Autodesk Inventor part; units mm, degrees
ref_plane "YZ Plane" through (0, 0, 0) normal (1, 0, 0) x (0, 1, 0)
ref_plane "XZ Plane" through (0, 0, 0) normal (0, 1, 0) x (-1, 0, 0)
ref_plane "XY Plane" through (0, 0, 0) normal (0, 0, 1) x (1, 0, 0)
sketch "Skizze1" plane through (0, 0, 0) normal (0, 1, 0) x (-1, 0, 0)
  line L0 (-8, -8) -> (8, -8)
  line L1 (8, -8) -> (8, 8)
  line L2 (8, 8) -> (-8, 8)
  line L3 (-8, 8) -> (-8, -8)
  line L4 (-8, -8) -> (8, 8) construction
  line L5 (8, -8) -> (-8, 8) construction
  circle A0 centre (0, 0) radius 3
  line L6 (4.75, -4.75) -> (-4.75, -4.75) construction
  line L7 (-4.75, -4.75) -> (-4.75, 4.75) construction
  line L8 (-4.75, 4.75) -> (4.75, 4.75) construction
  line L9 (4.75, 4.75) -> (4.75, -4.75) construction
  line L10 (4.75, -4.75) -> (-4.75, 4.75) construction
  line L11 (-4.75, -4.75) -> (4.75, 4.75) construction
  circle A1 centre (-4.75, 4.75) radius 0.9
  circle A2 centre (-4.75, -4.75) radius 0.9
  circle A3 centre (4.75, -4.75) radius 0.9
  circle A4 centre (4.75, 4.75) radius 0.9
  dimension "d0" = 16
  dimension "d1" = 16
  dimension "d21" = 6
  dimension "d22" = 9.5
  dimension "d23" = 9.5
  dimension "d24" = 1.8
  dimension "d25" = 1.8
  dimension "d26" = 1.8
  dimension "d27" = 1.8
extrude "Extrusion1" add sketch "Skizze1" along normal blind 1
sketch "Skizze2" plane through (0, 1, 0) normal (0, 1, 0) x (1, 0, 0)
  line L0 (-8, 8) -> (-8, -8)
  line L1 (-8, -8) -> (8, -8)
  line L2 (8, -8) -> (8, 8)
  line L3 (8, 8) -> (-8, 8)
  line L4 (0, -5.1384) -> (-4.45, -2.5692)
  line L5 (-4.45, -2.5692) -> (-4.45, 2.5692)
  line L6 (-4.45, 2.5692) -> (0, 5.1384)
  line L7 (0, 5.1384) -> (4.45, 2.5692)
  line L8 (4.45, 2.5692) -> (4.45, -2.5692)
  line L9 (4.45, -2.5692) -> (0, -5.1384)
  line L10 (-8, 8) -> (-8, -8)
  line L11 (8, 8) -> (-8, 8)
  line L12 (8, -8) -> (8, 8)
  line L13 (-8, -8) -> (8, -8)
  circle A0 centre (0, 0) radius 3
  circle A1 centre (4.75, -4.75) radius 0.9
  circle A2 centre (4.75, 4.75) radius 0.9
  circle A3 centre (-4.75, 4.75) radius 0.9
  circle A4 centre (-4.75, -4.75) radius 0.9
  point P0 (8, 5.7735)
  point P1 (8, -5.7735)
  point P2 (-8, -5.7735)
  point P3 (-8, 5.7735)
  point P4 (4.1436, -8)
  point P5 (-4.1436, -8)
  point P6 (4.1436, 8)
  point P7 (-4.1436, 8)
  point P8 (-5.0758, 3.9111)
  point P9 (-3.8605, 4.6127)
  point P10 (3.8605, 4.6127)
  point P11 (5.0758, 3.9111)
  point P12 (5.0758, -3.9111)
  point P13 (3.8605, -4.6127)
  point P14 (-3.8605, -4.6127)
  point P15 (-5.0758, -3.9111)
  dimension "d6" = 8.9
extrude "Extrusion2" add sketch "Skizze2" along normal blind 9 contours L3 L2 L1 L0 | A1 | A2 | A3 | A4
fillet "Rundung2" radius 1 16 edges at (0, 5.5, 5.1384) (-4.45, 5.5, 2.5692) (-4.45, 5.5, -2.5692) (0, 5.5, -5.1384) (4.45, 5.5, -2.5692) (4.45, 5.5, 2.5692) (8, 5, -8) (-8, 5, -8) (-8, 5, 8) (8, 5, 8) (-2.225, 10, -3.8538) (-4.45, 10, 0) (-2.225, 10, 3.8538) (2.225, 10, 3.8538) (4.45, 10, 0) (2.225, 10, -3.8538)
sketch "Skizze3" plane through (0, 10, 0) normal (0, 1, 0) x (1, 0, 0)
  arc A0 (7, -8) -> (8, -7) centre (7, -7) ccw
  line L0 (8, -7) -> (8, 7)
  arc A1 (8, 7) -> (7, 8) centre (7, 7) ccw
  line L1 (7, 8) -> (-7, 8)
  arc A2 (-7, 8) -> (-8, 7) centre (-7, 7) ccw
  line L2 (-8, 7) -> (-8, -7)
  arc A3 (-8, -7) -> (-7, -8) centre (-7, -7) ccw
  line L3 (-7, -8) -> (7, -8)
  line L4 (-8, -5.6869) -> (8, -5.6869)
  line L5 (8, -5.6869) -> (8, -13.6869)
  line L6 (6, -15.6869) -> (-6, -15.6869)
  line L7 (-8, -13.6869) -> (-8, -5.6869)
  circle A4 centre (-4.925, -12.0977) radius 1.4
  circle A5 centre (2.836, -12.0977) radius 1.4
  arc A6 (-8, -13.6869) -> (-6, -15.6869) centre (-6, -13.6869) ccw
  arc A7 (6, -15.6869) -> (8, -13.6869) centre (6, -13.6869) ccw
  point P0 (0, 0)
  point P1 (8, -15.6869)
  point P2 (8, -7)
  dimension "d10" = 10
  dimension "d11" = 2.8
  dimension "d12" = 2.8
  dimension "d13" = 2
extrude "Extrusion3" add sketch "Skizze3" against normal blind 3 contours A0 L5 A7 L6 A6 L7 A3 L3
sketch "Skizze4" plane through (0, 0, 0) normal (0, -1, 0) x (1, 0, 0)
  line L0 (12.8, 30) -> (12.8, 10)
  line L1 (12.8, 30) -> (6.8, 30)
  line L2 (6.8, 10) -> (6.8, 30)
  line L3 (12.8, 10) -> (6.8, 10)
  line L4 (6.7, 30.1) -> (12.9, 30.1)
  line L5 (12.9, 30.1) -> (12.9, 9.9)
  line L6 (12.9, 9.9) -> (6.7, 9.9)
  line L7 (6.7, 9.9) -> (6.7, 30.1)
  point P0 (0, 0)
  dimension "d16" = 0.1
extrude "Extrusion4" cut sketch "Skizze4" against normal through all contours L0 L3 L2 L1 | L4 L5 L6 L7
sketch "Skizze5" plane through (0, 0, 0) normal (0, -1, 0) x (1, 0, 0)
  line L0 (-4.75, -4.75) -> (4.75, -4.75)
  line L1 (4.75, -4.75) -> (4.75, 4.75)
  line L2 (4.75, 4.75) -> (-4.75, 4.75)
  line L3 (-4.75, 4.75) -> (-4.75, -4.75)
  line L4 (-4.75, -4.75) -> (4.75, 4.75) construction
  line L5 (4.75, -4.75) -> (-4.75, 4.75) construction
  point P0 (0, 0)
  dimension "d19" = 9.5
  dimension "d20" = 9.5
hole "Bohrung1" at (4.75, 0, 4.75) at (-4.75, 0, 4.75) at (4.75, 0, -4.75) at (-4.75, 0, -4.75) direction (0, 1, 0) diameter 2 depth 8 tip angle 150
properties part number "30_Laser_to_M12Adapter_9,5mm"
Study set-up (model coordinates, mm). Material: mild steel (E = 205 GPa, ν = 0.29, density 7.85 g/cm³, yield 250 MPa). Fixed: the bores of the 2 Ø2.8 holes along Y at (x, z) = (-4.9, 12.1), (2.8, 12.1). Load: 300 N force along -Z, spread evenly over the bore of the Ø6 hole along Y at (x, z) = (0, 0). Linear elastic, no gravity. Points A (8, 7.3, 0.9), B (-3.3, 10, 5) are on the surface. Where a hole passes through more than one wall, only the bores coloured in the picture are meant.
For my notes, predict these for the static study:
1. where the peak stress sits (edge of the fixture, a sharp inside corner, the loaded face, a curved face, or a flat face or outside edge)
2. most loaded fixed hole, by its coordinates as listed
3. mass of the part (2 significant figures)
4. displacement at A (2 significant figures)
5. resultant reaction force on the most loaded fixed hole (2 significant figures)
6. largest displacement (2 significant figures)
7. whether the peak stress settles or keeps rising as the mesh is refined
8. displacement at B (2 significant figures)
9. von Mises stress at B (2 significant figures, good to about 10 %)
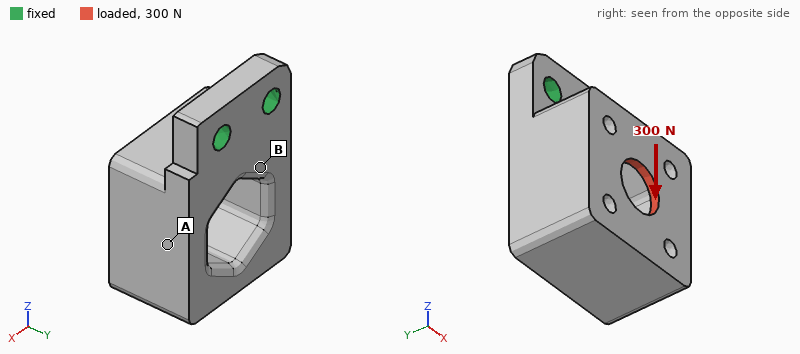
edge of the fixture
(2.8, 12.1)
17 g
14 µm
180 N
34 µm
keeps rising
6.9 µm
24 MPa
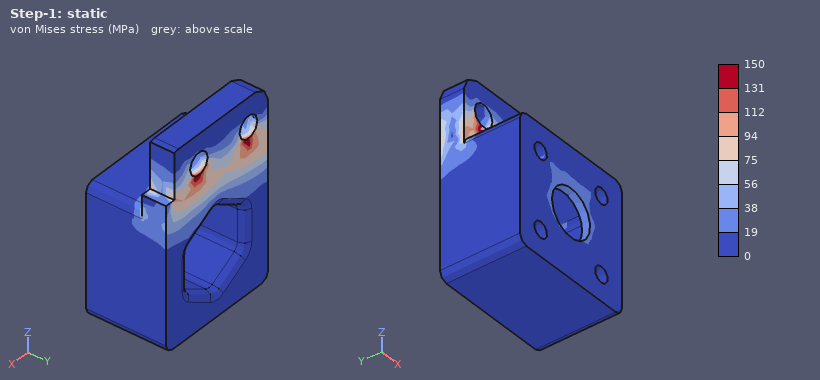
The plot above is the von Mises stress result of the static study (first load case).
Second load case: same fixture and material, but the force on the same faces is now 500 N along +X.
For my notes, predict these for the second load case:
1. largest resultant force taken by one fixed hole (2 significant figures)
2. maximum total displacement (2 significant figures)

750 N
12 µm
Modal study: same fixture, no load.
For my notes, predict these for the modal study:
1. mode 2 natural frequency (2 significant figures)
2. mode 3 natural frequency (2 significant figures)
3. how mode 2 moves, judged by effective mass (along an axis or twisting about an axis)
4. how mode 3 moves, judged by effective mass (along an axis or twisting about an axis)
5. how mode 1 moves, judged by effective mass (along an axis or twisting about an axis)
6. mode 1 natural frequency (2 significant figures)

12 kHz
15 kHz
along X
twisting about Z
along Y
4300 Hz
